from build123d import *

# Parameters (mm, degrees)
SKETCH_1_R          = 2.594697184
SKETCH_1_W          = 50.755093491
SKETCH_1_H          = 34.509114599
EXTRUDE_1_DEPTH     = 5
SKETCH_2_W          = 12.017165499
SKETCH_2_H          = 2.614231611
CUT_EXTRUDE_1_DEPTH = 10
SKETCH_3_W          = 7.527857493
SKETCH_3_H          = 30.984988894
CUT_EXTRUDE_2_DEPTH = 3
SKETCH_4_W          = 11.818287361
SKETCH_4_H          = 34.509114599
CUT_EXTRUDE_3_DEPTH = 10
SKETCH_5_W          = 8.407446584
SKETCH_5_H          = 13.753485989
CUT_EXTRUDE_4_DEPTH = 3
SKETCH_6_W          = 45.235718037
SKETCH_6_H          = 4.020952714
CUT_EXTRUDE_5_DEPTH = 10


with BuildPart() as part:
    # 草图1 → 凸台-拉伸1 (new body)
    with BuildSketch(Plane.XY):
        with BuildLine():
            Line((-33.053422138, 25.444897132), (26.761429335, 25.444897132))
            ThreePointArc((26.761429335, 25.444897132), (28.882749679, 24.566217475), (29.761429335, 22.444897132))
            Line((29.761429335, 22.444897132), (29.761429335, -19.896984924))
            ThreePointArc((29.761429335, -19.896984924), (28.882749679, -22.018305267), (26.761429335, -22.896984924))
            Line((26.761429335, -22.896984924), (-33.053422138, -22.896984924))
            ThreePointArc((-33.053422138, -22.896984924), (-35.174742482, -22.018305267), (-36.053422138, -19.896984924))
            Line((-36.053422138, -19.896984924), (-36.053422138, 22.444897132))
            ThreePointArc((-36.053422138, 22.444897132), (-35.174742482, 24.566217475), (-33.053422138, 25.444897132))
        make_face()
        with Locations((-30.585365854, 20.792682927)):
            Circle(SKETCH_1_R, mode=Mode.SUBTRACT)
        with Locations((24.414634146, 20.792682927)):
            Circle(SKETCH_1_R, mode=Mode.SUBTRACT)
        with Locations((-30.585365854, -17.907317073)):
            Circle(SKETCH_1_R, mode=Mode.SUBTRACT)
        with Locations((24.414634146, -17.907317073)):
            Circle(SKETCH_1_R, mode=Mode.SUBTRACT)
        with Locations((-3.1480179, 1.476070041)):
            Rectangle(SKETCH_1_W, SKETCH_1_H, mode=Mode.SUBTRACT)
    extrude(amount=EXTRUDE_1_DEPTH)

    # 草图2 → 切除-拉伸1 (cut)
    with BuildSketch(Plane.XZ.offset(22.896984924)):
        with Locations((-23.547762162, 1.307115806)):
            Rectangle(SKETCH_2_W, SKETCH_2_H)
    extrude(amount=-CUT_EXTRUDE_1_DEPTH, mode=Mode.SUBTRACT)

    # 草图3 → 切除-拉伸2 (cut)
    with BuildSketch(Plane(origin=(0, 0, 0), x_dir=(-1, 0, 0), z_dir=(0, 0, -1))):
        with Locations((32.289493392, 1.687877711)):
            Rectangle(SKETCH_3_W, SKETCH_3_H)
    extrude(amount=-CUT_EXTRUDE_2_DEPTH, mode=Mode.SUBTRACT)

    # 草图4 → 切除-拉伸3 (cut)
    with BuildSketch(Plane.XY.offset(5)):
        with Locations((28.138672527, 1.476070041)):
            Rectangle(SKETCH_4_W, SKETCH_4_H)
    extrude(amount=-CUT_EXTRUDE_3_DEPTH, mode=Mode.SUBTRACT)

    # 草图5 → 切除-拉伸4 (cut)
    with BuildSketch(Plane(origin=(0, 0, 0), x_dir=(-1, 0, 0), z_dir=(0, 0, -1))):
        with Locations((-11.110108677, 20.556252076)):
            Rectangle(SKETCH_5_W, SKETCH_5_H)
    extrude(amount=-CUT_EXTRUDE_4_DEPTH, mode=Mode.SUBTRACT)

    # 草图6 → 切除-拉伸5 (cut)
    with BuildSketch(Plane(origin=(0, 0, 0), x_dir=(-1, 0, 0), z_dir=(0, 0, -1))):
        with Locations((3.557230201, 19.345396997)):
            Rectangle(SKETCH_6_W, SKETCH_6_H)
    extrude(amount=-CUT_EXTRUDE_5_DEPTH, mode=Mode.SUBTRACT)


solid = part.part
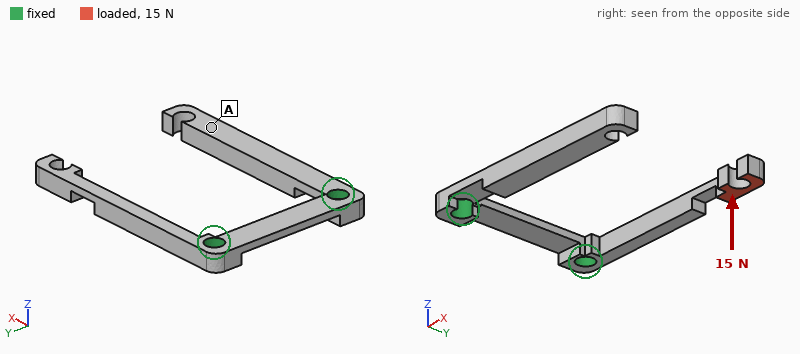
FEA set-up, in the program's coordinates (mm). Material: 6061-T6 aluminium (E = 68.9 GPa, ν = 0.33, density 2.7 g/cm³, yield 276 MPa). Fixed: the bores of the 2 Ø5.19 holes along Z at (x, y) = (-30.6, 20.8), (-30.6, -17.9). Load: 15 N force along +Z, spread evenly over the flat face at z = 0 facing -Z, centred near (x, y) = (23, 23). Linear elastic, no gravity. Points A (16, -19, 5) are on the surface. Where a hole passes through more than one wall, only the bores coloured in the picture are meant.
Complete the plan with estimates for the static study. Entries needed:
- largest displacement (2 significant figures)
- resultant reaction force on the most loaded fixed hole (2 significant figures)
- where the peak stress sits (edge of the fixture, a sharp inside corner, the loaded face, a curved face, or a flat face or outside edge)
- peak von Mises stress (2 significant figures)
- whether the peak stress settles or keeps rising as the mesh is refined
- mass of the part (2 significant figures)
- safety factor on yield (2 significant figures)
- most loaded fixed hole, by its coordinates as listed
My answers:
0.46 mm
15 N
a flat face or outside edge
78 MPa
settles
10 g
3.5
(-30.6, 20.8)
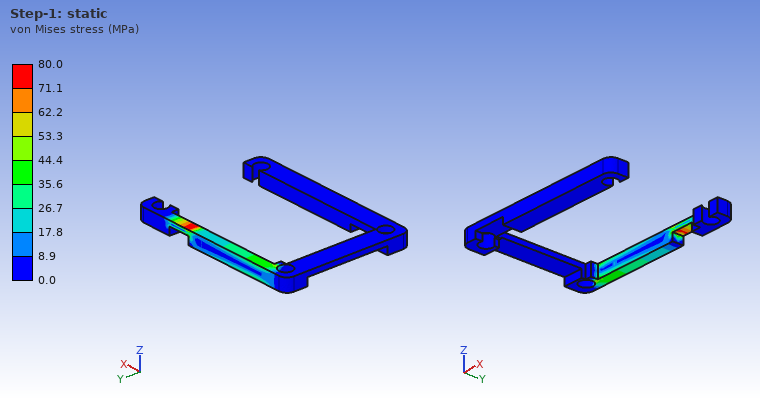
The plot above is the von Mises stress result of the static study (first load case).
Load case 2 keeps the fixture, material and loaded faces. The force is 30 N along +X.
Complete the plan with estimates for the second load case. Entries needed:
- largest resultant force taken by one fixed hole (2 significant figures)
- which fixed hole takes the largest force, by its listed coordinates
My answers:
30 N
(-30.6, 20.8)
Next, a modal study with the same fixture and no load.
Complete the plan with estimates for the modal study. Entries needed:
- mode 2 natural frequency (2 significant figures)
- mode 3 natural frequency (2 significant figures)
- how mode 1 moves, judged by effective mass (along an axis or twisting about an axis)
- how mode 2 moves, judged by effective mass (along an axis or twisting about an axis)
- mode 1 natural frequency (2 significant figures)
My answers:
990 Hz
1000 Hz
along Z
along Y
530 Hz
